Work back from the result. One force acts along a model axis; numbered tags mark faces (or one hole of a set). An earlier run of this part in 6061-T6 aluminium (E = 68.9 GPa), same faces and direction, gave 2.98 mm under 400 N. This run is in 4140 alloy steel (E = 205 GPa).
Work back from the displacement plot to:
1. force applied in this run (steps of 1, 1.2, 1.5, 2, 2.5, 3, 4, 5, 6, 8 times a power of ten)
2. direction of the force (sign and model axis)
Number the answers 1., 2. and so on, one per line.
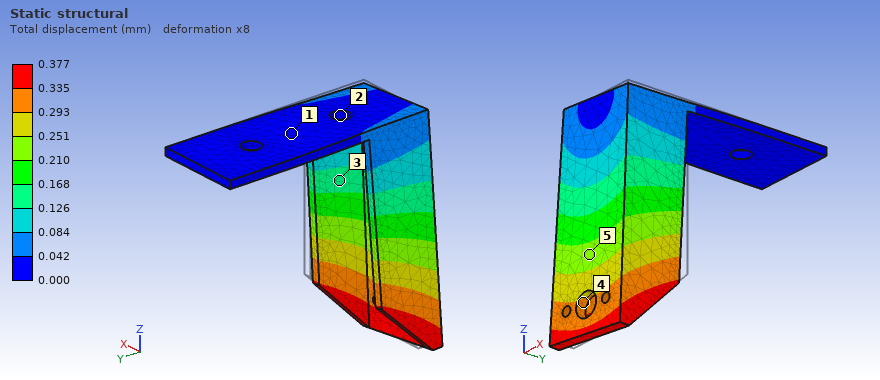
1. 150 N
2. -X
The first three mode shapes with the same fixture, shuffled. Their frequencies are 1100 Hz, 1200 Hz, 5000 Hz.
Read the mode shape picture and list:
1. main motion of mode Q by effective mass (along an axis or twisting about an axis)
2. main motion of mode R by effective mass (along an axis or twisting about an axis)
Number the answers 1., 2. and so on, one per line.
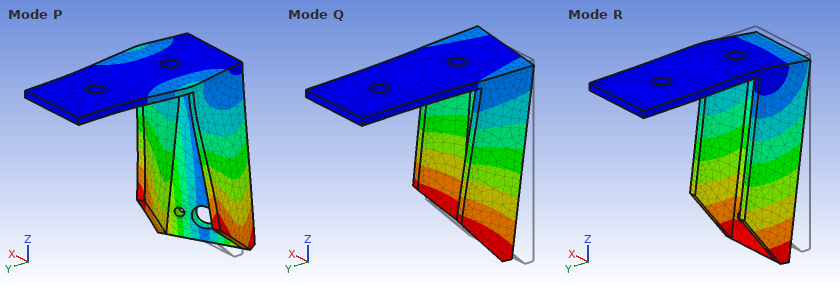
1. along X
2. along Y
